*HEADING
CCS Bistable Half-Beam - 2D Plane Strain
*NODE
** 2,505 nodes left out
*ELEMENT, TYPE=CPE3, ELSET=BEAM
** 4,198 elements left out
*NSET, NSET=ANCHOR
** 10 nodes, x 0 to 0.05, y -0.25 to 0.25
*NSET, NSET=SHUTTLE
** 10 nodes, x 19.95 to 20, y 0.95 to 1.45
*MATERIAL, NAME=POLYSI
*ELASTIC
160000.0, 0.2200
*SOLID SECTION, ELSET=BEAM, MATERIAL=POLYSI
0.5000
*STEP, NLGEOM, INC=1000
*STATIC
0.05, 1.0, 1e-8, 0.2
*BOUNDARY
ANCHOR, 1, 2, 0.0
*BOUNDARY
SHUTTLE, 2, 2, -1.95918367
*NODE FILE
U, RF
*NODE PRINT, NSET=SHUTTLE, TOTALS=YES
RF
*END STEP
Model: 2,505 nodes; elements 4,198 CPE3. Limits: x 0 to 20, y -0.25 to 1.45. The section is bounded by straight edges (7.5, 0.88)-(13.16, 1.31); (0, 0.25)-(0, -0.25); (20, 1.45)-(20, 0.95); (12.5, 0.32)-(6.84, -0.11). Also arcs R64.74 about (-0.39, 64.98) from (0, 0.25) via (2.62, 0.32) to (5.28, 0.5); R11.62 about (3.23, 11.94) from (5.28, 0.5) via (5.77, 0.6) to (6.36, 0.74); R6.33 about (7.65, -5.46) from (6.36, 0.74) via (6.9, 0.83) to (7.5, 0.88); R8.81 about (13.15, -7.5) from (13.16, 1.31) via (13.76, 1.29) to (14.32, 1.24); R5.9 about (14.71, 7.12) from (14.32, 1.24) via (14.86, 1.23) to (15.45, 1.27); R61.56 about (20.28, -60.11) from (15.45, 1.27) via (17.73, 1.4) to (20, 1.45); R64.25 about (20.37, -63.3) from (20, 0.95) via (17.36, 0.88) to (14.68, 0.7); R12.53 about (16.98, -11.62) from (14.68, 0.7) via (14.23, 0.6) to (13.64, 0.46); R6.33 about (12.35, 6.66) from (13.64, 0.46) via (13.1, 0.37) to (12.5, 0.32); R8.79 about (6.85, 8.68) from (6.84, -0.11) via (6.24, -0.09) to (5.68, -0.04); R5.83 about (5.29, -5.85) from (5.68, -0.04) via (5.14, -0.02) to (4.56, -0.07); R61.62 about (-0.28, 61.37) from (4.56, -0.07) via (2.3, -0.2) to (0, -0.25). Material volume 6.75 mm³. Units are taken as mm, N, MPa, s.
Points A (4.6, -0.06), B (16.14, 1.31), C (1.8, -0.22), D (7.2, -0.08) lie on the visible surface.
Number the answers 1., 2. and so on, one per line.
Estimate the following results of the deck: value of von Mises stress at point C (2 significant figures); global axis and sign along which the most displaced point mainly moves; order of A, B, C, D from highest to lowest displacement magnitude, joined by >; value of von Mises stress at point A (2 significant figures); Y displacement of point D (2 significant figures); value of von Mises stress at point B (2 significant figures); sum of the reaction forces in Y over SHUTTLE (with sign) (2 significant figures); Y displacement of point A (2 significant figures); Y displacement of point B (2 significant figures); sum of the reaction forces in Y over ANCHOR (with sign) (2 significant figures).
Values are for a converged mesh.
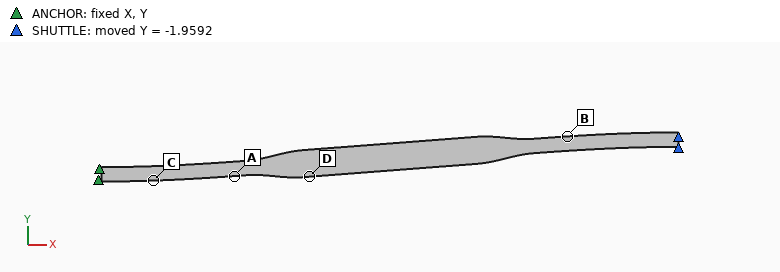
1. 840 MPa
2. -Y
3. B > D > A > C
4. 630 MPa
5. -0.53 mm
6. 270 MPa
7. -1.8 N
8. -0.24 mm
9. -1.6 mm
10. 1.8 N
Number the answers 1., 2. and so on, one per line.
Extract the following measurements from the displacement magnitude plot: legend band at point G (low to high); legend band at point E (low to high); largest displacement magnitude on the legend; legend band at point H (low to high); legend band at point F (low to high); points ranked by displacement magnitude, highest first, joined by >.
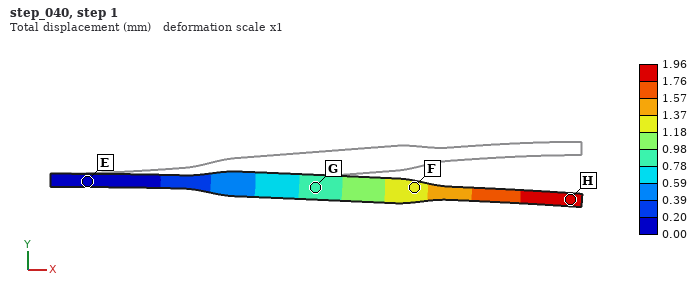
1. 0.78 to 0.98 mm
2. 0.00 to 0.20 mm
3. 1.96 mm
4. 1.76 to 1.96 mm
5. 1.18 to 1.37 mm
6. H > F > G > E
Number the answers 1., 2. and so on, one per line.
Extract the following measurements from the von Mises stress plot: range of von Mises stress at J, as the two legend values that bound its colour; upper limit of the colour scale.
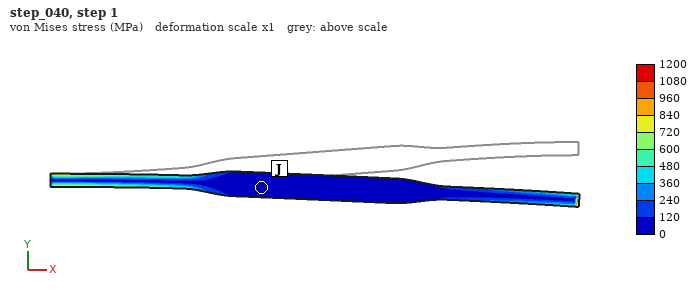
1. 0 to 120 MPa
2. 1200 MPa
